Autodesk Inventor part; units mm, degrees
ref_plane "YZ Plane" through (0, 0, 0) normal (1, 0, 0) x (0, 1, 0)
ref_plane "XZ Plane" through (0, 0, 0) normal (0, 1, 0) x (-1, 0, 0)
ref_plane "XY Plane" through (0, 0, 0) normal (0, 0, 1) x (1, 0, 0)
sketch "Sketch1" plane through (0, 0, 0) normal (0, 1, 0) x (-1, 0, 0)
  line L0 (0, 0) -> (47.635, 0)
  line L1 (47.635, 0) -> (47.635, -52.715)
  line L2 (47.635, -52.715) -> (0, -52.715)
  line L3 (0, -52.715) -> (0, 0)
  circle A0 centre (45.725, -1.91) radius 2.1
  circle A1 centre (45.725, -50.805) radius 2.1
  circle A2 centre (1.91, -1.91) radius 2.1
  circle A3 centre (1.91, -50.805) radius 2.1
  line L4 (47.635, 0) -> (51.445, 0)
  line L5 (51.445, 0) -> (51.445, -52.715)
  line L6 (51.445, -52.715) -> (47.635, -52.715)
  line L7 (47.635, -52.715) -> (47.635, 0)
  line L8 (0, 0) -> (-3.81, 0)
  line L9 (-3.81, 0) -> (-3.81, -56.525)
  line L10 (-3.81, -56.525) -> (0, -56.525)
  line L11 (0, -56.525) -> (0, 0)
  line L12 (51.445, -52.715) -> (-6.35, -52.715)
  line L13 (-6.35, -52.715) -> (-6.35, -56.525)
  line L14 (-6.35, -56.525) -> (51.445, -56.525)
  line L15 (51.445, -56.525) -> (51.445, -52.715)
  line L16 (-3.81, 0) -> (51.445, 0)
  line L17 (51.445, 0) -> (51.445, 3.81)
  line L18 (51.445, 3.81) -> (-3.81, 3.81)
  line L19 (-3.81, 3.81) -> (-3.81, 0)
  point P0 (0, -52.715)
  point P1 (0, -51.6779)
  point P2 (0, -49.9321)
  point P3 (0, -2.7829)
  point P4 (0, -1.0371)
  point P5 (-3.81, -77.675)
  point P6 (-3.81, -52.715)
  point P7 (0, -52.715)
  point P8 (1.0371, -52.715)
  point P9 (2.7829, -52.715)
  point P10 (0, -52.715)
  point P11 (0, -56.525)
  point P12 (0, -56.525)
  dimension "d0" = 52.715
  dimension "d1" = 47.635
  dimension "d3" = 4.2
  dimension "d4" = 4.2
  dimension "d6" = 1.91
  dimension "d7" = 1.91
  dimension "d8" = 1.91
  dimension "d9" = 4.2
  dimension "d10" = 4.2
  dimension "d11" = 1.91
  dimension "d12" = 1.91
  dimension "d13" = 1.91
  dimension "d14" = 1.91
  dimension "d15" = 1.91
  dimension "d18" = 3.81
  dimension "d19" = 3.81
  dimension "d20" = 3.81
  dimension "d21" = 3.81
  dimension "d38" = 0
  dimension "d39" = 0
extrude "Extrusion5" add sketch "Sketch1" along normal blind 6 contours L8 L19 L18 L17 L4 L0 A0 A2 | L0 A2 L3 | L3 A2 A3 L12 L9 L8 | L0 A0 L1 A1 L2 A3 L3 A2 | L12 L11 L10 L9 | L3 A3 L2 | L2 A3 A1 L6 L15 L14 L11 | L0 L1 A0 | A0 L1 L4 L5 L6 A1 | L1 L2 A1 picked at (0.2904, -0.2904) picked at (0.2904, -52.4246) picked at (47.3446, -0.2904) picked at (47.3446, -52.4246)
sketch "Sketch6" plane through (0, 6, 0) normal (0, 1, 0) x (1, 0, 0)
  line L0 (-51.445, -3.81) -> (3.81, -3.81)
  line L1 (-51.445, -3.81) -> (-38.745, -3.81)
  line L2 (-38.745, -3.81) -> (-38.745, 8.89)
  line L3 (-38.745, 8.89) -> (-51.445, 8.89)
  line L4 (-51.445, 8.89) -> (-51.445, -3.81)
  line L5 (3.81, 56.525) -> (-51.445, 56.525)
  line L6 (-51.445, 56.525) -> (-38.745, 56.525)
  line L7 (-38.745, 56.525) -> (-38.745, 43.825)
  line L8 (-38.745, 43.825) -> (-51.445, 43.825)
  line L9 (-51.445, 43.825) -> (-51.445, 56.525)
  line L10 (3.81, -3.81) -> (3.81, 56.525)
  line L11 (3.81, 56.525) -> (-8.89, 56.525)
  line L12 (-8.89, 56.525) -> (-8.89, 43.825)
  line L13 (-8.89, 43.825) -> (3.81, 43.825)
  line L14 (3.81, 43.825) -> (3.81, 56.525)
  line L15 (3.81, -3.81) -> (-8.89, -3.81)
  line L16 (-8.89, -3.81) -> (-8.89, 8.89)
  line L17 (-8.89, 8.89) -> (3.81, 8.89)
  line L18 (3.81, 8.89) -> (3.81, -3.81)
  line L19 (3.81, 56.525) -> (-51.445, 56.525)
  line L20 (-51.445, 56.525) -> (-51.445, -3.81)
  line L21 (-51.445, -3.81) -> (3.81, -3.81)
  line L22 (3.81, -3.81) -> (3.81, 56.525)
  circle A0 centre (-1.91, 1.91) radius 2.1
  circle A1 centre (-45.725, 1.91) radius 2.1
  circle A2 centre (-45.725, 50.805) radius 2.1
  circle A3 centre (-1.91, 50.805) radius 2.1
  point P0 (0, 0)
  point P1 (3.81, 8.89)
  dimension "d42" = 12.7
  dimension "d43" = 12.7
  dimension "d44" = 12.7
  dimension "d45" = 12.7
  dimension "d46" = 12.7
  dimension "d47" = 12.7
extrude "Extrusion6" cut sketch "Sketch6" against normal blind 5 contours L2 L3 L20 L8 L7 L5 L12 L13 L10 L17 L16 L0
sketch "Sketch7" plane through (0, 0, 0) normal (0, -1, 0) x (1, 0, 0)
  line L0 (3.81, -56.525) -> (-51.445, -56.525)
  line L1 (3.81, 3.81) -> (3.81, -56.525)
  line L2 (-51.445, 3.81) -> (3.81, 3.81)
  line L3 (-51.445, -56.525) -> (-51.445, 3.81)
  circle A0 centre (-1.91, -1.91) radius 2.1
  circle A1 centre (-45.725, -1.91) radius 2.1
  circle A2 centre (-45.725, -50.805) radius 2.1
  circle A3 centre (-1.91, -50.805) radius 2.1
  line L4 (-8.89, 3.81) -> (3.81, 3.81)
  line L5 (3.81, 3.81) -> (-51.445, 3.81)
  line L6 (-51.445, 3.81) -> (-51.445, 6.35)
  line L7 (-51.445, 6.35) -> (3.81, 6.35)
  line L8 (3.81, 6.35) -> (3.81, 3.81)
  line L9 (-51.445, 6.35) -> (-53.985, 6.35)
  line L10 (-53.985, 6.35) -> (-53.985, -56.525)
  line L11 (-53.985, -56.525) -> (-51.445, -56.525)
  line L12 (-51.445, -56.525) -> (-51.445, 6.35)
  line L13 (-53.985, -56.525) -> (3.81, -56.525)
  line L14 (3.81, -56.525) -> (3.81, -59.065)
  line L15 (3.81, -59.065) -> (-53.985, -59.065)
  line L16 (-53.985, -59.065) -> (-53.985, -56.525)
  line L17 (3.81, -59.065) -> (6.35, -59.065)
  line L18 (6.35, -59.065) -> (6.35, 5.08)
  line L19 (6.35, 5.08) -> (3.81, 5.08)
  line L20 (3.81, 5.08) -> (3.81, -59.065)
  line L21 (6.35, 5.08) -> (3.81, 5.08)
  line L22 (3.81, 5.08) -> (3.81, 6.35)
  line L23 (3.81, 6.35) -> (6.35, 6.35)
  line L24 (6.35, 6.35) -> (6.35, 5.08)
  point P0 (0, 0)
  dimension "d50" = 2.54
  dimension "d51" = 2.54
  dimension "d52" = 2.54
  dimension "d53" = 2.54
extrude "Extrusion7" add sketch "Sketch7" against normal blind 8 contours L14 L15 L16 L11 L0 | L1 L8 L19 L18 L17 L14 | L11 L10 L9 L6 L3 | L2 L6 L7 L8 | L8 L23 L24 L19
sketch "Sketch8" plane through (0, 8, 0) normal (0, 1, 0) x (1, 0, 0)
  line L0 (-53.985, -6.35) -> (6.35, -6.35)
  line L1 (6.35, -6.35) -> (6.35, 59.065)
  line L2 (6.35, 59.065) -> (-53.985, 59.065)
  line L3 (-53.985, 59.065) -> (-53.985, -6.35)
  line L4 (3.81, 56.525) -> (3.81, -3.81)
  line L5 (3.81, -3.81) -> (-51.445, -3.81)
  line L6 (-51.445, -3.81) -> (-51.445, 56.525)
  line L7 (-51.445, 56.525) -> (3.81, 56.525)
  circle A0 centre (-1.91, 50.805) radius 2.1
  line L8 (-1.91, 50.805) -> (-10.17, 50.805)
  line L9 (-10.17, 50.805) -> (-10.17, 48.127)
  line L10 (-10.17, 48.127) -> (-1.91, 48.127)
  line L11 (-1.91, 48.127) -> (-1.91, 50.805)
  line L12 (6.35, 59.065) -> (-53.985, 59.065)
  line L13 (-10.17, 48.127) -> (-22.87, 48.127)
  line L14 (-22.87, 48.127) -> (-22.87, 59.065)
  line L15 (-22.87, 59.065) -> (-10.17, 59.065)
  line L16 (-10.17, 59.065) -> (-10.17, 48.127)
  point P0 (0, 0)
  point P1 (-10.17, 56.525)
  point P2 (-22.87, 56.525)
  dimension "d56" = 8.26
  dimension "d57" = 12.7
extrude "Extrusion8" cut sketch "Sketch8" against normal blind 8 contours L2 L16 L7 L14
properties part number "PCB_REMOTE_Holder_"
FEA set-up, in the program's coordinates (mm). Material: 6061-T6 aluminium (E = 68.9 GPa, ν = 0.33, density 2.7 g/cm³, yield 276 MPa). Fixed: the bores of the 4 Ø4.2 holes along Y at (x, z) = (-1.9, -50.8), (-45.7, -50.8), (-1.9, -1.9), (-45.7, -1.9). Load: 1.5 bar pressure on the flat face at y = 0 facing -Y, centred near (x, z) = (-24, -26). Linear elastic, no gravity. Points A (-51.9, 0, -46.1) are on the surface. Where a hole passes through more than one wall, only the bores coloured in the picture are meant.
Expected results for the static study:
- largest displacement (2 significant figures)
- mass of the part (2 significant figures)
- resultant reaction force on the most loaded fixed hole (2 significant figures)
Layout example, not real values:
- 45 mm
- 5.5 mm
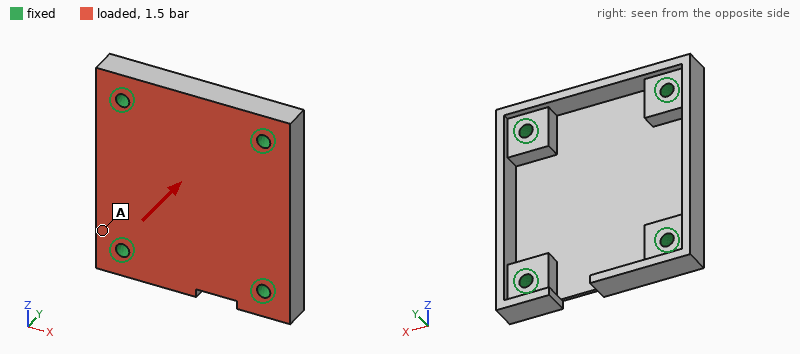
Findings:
- 0.19 mm
- 29 g
- 180 N
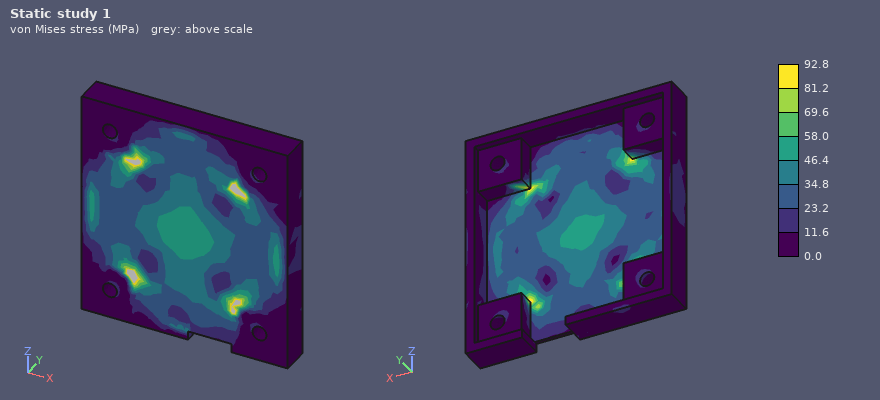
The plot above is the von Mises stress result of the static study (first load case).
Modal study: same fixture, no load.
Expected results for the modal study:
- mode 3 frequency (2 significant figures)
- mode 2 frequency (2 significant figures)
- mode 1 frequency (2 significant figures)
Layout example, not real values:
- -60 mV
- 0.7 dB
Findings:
- 6800 Hz
- 6700 Hz
- 3500 Hz
